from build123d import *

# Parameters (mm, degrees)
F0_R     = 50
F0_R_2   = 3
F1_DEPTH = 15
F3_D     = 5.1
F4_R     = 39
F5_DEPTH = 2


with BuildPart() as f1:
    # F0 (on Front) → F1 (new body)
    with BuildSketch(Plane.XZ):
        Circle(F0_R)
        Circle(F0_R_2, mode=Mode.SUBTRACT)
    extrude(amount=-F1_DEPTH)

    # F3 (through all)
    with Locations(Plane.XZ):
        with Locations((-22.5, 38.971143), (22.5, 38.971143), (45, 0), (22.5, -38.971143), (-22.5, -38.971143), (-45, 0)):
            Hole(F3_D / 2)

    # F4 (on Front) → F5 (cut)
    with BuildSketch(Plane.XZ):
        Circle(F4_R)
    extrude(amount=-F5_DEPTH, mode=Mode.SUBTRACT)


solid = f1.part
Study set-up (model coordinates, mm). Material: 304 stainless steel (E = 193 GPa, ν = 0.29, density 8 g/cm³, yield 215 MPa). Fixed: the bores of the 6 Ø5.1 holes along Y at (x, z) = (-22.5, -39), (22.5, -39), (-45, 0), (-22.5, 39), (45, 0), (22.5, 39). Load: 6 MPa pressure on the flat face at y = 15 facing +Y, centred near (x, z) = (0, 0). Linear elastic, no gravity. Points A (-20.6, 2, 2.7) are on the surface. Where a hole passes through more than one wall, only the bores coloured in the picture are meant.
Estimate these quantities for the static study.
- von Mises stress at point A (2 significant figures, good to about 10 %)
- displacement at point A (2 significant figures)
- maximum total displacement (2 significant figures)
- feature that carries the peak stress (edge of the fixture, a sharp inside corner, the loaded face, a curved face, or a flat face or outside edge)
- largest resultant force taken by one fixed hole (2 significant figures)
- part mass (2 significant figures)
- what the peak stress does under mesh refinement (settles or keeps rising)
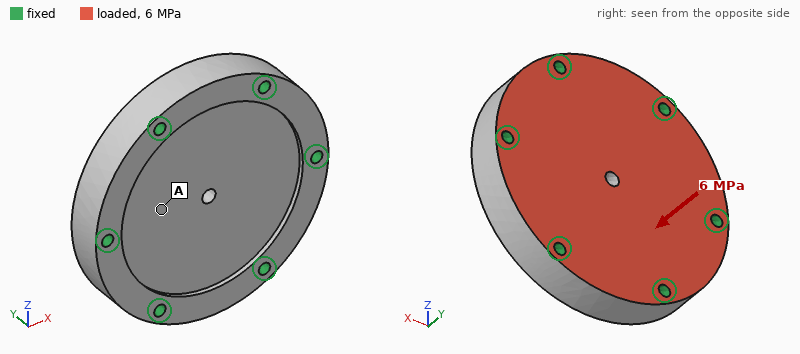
25 MPa
14 µm
19 µm
edge of the fixture
7.8 kN
850 g
keeps rising
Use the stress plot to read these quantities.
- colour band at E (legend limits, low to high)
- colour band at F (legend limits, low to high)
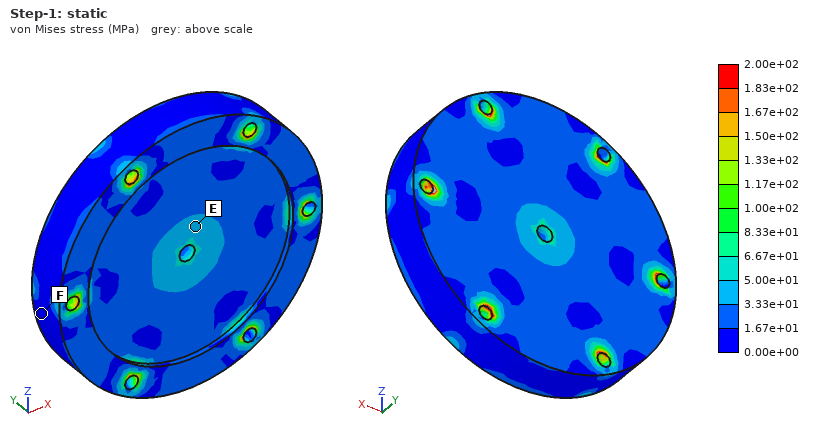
3.33e+01 to 5.00e+01 MPa
0.00e+00 to 1.67e+01 MPa
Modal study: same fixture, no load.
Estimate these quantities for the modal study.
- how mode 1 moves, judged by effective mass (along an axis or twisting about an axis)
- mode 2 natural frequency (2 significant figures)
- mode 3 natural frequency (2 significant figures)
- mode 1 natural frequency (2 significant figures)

along Y
19 kHz
19 kHz
11 kHz
